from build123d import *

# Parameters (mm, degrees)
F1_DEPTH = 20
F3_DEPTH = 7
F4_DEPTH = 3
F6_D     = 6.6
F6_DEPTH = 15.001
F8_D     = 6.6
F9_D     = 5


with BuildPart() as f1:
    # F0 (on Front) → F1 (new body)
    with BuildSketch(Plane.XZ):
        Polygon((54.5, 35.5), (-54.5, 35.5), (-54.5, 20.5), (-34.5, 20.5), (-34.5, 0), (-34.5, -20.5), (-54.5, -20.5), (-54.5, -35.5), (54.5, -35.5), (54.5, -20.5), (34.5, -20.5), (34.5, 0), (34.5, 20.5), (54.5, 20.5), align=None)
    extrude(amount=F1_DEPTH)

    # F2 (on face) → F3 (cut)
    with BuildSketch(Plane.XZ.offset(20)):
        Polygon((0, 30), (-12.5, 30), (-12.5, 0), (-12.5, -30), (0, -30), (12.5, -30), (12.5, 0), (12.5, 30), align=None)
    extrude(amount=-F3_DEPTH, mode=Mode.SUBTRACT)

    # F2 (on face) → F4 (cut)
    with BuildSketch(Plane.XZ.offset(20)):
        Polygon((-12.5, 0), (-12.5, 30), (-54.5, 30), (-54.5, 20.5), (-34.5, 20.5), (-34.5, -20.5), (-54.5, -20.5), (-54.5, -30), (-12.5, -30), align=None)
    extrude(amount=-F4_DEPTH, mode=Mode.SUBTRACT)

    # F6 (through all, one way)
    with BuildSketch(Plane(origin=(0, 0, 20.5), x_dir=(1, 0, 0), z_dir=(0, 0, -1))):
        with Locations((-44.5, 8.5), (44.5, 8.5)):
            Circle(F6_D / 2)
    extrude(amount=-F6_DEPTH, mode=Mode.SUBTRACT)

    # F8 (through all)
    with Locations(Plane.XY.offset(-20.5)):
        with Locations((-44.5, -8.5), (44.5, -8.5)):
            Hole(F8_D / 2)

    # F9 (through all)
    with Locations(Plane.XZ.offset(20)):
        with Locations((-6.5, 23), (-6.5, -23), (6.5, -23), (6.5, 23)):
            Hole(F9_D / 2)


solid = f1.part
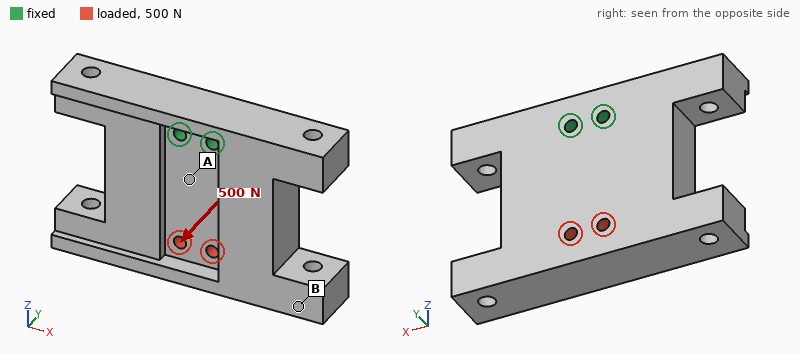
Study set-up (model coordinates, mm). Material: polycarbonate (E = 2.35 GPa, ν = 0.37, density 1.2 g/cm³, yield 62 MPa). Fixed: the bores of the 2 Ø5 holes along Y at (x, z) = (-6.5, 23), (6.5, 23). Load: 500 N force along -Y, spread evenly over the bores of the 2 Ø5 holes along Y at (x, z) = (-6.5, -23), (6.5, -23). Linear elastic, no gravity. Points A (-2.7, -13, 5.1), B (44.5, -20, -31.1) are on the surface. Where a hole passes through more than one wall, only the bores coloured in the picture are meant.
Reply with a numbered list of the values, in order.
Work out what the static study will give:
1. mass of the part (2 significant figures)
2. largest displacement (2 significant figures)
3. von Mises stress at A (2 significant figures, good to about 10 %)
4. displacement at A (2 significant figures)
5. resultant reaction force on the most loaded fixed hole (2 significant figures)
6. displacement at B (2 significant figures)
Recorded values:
1. 120 g
2. 0.80 mm
3. 4.6 MPa
4. 0.18 mm
5. 260 N
6. 0.66 mm
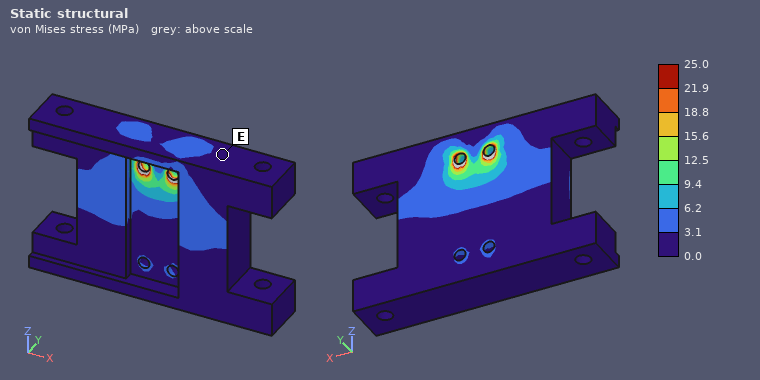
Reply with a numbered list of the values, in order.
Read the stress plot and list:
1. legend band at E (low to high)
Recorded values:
1. 0.0 to 3.1 MPa
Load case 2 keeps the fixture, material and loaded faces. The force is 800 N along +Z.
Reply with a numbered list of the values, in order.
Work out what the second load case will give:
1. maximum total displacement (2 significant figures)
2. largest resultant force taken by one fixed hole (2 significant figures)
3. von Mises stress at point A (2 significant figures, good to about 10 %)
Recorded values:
1. 43 µm
2. 400 N
3. 1.8 MPa
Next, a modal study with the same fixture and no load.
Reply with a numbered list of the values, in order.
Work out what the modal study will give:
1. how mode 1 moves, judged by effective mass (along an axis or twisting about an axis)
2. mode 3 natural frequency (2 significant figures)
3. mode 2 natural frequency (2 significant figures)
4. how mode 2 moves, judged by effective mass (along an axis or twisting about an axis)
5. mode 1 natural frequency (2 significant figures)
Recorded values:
1. along Y
2. 790 Hz
3. 730 Hz
4. along X
5. 590 Hz
